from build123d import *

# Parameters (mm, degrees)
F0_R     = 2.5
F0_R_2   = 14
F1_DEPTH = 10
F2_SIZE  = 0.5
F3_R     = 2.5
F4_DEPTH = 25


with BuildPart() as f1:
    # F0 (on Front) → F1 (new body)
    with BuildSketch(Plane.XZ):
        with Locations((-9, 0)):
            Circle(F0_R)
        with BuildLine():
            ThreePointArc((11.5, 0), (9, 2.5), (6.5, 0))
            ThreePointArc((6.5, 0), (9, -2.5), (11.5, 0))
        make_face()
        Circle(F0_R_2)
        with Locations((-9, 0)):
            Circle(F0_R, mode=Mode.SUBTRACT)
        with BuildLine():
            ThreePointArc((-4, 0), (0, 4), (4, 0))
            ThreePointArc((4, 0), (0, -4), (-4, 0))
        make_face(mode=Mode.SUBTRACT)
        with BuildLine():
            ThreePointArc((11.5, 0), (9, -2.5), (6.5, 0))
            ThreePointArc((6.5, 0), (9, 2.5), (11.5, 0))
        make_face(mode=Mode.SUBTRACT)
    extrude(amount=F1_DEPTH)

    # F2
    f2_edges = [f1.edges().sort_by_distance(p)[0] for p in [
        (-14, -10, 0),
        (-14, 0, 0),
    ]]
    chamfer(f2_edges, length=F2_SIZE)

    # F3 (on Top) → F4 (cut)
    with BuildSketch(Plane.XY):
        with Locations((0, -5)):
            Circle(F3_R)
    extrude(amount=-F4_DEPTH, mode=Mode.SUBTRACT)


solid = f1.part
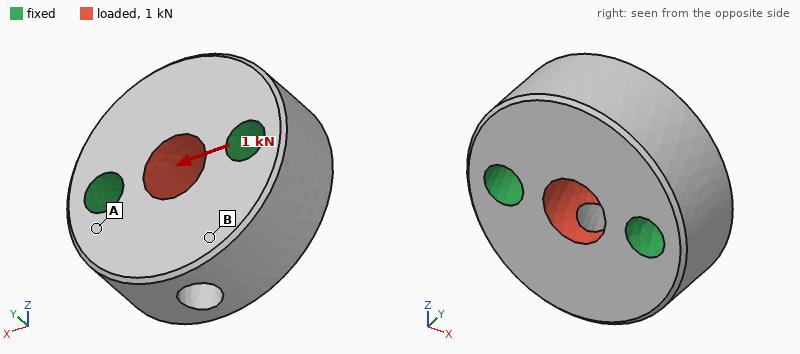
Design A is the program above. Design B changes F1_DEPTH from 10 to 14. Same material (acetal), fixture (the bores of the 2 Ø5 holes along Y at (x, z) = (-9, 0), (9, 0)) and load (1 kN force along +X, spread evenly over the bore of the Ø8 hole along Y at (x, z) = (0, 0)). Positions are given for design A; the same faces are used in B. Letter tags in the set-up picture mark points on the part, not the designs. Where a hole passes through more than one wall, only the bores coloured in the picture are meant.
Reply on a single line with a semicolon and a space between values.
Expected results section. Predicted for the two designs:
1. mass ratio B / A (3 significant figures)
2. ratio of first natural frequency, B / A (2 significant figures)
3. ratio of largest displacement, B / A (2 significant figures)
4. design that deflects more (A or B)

1.42; 1.2; 0.69; A
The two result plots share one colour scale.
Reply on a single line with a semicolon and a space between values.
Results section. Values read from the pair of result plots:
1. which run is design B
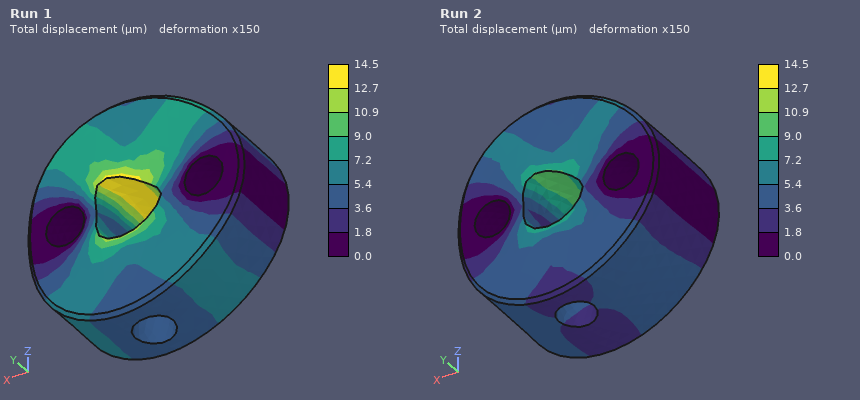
Run 2
